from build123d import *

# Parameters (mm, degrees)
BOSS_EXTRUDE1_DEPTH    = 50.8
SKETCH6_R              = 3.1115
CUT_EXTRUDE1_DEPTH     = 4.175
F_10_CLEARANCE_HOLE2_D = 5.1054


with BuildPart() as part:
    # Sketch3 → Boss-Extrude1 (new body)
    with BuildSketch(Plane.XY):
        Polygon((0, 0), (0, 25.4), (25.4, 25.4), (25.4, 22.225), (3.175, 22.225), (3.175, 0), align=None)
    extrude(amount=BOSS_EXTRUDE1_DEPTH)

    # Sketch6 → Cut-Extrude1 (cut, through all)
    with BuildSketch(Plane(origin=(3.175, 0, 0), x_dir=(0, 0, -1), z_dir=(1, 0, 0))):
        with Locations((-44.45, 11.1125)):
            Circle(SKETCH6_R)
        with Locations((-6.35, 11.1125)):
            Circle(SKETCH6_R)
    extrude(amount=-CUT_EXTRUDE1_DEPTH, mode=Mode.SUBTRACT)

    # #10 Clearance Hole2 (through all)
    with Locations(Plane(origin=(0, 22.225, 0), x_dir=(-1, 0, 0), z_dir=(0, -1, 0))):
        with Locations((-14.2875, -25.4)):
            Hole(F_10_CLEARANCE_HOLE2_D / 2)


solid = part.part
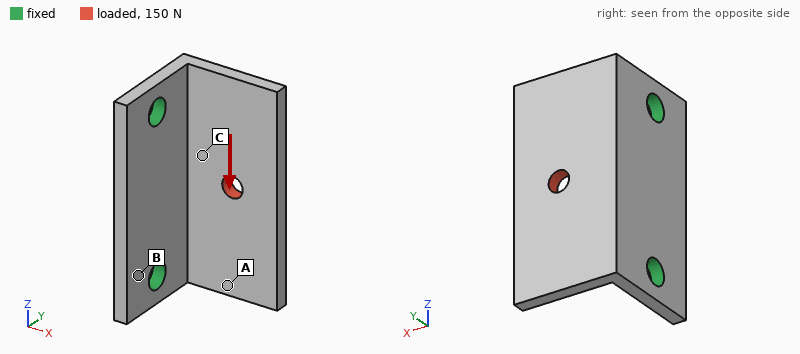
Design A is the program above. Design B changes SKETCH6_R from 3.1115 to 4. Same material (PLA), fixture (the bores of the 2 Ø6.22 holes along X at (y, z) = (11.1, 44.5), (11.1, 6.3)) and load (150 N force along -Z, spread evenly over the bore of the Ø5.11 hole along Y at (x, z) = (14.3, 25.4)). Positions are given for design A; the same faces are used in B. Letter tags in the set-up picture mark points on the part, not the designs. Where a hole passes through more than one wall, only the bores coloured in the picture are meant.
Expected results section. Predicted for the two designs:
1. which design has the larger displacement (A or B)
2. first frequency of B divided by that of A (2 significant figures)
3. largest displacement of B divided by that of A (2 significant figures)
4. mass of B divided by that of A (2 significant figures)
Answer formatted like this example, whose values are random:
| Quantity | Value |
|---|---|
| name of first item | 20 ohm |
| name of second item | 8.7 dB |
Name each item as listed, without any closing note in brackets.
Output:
| Quantity | Value |
|---|---|
| which design has the larger displacement | A |
| first frequency of B divided by that of A | 1.1 |
| largest displacement of B divided by that of A | 0.84 |
| mass of B divided by that of A | 0.98 |
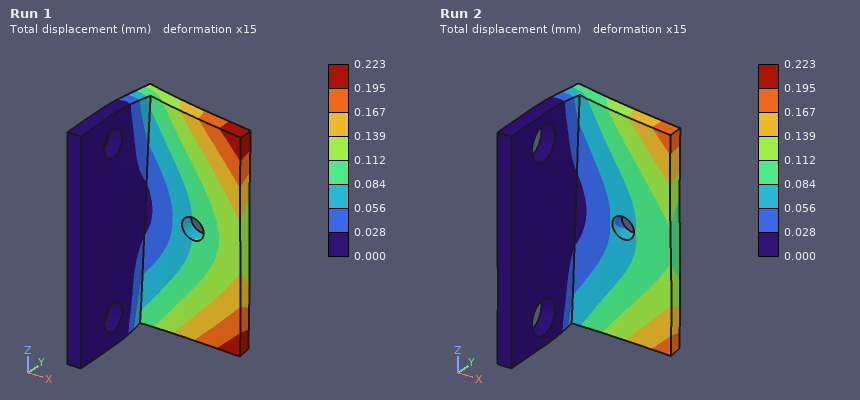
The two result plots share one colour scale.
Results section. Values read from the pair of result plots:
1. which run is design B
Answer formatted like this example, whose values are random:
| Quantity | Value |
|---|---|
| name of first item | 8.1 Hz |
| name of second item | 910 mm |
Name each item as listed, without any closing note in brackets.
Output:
| Quantity | Value |
|---|---|
| which run is design B | Run 2 |
